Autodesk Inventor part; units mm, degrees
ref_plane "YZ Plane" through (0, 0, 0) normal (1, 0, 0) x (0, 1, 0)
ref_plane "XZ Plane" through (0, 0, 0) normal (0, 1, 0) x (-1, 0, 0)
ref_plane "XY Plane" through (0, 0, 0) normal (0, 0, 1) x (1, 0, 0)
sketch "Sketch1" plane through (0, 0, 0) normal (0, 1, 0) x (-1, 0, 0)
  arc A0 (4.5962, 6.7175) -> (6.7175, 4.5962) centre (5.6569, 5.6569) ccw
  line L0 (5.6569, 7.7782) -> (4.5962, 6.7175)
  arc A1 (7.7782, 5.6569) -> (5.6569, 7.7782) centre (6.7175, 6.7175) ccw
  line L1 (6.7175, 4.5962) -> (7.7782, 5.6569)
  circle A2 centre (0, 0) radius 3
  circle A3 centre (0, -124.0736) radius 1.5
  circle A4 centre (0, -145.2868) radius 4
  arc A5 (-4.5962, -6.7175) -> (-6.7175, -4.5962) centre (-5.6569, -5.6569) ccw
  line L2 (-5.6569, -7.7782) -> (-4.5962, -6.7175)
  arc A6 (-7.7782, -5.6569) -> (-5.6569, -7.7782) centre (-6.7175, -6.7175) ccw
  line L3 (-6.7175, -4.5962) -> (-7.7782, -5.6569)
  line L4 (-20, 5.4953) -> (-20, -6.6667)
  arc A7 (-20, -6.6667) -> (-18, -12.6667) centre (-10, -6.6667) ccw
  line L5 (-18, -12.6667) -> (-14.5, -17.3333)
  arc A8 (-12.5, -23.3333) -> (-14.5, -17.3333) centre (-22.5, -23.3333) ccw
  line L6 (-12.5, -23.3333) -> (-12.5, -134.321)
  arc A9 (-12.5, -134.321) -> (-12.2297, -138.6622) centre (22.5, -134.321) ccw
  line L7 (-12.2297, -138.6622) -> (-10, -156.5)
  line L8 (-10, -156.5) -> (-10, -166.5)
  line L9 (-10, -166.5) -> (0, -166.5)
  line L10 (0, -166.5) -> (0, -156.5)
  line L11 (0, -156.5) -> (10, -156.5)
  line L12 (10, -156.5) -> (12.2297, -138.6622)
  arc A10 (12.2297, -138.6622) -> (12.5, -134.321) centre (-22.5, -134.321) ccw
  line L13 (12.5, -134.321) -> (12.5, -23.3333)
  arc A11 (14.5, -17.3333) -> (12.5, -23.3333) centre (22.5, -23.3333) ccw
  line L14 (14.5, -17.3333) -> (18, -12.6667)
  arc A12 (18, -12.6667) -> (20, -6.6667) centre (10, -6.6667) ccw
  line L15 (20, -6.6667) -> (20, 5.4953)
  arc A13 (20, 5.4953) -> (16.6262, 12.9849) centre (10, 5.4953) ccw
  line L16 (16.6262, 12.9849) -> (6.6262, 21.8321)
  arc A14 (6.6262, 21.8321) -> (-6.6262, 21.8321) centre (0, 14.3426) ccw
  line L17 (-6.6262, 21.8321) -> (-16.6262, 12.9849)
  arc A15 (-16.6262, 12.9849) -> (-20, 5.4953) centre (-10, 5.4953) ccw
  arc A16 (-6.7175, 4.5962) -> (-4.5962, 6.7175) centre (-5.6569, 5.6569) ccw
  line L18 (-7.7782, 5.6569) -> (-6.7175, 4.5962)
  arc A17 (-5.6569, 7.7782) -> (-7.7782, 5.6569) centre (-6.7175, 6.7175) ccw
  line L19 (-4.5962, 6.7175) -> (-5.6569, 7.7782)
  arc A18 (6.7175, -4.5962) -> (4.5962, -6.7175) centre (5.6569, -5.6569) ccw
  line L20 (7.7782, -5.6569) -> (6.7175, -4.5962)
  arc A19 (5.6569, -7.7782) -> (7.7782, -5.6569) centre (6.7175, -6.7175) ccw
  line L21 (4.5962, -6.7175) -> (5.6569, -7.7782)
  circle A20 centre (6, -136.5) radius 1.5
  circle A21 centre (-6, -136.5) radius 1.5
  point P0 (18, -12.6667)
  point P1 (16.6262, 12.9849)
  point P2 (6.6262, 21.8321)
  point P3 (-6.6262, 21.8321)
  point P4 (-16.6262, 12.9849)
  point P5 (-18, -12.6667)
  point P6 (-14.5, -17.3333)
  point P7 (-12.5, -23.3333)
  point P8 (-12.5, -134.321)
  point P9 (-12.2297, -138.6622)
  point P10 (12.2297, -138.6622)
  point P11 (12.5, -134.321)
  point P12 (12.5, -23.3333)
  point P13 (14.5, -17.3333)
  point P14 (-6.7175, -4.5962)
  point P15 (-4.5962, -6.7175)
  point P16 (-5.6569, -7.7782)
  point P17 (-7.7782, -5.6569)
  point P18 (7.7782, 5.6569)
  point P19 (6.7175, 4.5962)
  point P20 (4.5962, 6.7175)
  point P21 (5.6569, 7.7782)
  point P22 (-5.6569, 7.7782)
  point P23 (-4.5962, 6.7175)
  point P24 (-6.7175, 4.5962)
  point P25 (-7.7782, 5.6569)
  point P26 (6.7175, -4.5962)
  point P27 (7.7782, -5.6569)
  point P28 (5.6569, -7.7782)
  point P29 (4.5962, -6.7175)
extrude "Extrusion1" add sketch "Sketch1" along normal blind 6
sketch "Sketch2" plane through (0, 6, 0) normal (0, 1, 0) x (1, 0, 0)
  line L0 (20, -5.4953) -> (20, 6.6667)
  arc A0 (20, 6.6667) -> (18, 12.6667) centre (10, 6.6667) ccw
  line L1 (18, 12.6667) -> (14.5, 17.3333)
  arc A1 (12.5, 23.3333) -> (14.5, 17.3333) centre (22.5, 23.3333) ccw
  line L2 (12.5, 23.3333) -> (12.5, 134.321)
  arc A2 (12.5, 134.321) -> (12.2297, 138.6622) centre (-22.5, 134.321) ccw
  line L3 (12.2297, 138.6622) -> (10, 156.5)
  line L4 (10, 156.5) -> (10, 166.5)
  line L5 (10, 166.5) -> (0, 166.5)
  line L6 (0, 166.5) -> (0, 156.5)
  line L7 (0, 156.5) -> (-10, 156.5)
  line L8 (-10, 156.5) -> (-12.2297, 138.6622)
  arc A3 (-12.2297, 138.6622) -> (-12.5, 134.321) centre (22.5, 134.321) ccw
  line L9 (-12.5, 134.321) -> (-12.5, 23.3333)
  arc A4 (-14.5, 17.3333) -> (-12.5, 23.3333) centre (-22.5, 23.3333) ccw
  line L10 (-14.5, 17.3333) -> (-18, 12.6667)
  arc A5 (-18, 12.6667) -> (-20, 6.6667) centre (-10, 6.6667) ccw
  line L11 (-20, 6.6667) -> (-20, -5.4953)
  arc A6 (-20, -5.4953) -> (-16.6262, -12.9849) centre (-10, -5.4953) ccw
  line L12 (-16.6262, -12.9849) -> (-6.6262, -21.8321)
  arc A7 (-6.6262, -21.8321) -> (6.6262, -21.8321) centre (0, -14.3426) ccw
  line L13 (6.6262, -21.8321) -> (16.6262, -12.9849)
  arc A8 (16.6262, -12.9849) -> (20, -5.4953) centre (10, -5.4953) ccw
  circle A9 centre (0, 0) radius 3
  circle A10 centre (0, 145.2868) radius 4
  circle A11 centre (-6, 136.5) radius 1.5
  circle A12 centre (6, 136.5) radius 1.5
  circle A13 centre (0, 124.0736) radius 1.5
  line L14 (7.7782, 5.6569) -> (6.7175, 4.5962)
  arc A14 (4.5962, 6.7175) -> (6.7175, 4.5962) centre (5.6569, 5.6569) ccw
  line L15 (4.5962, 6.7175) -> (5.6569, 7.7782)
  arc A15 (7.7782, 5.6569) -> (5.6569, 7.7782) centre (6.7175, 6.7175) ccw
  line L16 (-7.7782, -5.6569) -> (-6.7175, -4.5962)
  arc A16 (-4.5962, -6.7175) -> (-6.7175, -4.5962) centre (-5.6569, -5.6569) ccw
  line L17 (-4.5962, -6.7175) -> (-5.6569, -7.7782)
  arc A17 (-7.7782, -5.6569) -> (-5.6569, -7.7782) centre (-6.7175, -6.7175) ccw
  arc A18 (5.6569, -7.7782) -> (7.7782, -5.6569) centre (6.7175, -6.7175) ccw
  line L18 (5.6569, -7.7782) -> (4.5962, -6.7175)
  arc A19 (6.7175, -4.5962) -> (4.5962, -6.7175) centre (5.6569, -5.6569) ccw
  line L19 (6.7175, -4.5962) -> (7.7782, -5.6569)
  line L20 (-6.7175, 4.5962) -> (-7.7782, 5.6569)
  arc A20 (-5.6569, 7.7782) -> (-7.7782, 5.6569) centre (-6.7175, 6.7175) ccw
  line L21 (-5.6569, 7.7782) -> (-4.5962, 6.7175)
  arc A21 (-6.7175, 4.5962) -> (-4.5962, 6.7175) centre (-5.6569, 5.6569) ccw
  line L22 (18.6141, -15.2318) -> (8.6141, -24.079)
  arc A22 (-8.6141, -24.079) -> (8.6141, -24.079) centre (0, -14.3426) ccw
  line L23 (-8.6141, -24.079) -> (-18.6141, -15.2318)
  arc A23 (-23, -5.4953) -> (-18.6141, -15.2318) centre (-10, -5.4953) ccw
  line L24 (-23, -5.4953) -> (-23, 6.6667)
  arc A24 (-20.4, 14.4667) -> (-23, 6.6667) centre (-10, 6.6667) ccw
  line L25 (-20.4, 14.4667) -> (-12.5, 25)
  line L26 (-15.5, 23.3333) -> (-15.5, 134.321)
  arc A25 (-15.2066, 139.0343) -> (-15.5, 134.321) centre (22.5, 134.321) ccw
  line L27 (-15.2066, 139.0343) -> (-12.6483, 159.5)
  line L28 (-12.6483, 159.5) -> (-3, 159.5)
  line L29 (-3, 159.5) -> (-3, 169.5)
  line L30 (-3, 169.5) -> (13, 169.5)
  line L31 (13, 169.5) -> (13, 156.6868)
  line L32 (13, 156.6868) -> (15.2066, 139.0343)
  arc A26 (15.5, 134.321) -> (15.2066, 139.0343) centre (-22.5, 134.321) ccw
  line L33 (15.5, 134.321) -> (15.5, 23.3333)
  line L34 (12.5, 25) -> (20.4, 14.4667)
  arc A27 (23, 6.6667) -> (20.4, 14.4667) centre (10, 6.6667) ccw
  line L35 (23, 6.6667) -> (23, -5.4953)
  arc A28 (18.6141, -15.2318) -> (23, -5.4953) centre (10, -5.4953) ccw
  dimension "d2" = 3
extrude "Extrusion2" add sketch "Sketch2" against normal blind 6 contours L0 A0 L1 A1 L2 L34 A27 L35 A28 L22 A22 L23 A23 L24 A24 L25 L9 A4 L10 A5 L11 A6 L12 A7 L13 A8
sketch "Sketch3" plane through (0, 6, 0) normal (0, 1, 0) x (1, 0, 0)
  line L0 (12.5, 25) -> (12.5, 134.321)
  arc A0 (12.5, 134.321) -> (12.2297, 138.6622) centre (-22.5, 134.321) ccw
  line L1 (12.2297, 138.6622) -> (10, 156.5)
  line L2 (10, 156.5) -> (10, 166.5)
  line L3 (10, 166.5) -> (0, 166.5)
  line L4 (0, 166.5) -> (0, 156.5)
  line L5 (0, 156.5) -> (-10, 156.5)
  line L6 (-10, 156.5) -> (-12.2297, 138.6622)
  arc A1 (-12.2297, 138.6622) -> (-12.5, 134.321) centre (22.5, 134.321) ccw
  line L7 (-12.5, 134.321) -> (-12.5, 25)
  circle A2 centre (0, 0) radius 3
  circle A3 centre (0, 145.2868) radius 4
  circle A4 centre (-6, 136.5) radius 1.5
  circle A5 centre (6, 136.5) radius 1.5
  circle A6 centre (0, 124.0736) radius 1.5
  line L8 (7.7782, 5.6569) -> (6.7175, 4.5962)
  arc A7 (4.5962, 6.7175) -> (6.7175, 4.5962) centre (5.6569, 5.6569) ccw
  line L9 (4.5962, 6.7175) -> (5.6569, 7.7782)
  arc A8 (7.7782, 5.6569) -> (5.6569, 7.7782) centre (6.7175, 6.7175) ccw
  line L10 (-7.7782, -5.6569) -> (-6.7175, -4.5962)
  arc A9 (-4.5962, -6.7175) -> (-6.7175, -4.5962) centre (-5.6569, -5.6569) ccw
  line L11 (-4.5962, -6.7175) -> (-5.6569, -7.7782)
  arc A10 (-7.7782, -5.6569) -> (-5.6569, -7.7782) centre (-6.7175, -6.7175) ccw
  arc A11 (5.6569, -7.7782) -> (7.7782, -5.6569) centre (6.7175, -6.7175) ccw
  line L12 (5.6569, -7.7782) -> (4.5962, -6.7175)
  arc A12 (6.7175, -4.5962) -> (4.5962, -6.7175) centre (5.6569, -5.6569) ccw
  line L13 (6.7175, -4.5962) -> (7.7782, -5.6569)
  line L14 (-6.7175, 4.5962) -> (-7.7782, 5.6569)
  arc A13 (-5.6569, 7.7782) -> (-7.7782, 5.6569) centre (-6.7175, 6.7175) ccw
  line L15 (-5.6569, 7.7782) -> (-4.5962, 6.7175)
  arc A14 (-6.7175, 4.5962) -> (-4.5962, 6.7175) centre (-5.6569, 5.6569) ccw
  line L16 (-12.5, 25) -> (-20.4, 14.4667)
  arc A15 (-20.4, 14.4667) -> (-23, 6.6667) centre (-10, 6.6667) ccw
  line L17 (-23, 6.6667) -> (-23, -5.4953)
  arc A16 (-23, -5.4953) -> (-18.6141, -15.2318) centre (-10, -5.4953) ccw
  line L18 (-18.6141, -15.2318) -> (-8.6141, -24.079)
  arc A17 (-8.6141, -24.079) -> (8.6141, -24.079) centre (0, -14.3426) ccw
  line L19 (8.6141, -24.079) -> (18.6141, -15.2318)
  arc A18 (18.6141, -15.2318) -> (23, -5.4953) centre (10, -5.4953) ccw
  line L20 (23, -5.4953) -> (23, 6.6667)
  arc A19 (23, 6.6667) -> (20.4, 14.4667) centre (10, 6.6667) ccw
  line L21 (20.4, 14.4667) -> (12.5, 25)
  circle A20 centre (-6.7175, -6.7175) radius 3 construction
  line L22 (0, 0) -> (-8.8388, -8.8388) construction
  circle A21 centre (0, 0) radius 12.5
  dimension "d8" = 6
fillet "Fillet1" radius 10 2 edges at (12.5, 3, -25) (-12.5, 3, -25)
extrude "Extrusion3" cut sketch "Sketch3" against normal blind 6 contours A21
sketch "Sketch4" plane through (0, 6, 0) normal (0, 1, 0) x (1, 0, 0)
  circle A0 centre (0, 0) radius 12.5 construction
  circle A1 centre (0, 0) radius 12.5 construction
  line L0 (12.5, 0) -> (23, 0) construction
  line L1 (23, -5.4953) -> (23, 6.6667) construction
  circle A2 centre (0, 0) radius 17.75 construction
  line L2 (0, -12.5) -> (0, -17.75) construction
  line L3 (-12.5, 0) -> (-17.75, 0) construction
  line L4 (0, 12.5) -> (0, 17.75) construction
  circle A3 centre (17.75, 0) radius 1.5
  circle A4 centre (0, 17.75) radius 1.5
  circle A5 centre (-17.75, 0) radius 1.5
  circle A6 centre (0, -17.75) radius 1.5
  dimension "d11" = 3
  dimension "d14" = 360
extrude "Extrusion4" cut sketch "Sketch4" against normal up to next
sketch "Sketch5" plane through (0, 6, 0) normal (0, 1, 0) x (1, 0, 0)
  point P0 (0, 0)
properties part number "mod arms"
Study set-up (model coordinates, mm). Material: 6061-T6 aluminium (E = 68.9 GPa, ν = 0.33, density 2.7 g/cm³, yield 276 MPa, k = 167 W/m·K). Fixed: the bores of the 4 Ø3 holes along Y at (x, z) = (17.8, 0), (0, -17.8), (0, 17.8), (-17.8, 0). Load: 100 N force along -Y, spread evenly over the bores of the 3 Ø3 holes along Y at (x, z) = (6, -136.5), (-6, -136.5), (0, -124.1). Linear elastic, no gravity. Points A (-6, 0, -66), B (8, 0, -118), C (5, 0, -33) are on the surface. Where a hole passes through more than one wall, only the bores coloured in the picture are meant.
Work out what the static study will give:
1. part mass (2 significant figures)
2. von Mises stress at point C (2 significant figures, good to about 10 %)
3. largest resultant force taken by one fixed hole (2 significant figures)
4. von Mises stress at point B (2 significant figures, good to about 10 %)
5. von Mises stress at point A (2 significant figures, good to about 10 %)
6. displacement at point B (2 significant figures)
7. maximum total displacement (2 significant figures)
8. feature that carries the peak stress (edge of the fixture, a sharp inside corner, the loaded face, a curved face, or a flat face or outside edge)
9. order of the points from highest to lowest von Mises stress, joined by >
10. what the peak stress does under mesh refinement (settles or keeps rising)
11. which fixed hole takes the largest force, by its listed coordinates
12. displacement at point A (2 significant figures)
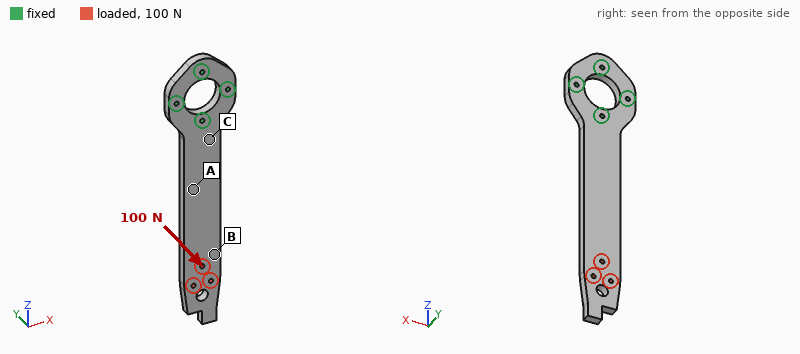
76 g
63 MPa
400 N
9.9 MPa
44 MPa
1.3 mm
2.4 mm
edge of the fixture
C > A > B
keeps rising
(0, -17.8)
0.38 mm
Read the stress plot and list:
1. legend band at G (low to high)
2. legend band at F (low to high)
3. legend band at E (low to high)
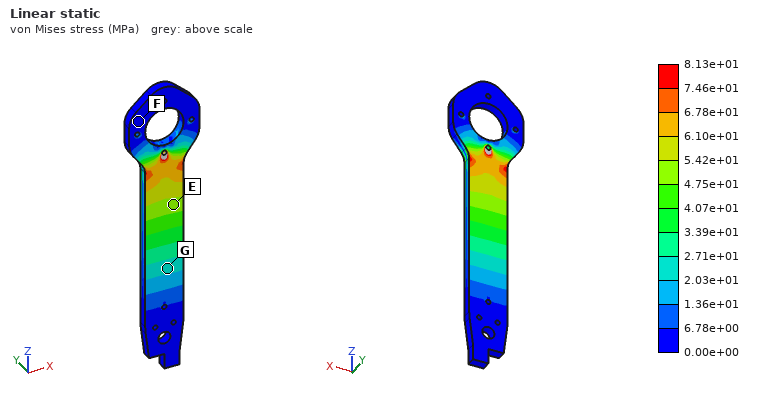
2.03e+01 to 2.71e+01 MPa
0.00e+00 to 6.78e+00 MPa
4.75e+01 to 5.42e+01 MPa
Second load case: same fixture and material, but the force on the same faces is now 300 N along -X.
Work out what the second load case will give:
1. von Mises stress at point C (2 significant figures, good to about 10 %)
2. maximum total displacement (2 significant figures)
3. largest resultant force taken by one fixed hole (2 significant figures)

18 MPa
0.46 mm
1.1 kN
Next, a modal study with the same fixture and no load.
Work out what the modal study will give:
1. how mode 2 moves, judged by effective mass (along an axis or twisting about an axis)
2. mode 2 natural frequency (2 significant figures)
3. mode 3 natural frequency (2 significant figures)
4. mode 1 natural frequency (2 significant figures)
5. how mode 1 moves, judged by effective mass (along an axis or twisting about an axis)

along X
970 Hz
1500 Hz
250 Hz
along Y
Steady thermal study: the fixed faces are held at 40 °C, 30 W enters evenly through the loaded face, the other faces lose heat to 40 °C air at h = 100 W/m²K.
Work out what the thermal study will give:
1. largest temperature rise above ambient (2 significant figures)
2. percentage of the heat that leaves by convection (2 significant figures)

51 K
78 %
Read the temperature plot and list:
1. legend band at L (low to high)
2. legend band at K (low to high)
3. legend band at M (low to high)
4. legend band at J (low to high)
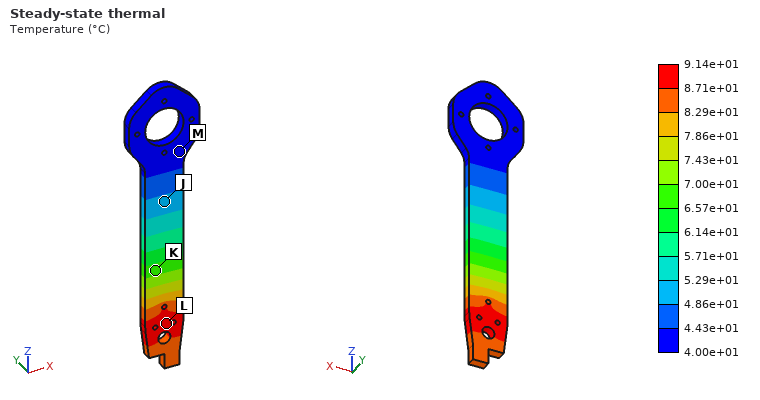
8.71e+01 to 9.14e+01 °C
6.57e+01 to 7.00e+01 °C
4.00e+01 to 4.43e+01 °C
4.86e+01 to 5.29e+01 °C
